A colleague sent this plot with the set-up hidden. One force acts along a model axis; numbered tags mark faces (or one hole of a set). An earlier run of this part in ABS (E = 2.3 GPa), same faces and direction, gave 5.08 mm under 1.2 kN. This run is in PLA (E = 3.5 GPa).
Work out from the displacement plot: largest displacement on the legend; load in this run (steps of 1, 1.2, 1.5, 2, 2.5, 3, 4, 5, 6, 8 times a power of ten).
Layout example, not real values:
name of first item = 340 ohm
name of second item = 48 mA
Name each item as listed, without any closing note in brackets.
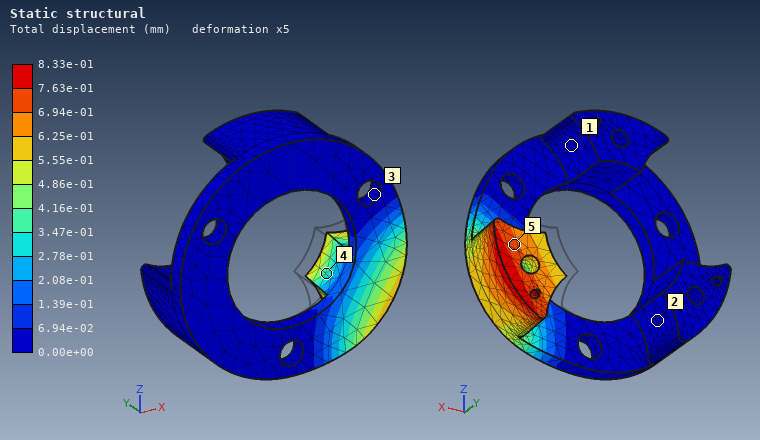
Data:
largest displacement on the legend = 8.33e-01 mm
load in this run = 300 N
